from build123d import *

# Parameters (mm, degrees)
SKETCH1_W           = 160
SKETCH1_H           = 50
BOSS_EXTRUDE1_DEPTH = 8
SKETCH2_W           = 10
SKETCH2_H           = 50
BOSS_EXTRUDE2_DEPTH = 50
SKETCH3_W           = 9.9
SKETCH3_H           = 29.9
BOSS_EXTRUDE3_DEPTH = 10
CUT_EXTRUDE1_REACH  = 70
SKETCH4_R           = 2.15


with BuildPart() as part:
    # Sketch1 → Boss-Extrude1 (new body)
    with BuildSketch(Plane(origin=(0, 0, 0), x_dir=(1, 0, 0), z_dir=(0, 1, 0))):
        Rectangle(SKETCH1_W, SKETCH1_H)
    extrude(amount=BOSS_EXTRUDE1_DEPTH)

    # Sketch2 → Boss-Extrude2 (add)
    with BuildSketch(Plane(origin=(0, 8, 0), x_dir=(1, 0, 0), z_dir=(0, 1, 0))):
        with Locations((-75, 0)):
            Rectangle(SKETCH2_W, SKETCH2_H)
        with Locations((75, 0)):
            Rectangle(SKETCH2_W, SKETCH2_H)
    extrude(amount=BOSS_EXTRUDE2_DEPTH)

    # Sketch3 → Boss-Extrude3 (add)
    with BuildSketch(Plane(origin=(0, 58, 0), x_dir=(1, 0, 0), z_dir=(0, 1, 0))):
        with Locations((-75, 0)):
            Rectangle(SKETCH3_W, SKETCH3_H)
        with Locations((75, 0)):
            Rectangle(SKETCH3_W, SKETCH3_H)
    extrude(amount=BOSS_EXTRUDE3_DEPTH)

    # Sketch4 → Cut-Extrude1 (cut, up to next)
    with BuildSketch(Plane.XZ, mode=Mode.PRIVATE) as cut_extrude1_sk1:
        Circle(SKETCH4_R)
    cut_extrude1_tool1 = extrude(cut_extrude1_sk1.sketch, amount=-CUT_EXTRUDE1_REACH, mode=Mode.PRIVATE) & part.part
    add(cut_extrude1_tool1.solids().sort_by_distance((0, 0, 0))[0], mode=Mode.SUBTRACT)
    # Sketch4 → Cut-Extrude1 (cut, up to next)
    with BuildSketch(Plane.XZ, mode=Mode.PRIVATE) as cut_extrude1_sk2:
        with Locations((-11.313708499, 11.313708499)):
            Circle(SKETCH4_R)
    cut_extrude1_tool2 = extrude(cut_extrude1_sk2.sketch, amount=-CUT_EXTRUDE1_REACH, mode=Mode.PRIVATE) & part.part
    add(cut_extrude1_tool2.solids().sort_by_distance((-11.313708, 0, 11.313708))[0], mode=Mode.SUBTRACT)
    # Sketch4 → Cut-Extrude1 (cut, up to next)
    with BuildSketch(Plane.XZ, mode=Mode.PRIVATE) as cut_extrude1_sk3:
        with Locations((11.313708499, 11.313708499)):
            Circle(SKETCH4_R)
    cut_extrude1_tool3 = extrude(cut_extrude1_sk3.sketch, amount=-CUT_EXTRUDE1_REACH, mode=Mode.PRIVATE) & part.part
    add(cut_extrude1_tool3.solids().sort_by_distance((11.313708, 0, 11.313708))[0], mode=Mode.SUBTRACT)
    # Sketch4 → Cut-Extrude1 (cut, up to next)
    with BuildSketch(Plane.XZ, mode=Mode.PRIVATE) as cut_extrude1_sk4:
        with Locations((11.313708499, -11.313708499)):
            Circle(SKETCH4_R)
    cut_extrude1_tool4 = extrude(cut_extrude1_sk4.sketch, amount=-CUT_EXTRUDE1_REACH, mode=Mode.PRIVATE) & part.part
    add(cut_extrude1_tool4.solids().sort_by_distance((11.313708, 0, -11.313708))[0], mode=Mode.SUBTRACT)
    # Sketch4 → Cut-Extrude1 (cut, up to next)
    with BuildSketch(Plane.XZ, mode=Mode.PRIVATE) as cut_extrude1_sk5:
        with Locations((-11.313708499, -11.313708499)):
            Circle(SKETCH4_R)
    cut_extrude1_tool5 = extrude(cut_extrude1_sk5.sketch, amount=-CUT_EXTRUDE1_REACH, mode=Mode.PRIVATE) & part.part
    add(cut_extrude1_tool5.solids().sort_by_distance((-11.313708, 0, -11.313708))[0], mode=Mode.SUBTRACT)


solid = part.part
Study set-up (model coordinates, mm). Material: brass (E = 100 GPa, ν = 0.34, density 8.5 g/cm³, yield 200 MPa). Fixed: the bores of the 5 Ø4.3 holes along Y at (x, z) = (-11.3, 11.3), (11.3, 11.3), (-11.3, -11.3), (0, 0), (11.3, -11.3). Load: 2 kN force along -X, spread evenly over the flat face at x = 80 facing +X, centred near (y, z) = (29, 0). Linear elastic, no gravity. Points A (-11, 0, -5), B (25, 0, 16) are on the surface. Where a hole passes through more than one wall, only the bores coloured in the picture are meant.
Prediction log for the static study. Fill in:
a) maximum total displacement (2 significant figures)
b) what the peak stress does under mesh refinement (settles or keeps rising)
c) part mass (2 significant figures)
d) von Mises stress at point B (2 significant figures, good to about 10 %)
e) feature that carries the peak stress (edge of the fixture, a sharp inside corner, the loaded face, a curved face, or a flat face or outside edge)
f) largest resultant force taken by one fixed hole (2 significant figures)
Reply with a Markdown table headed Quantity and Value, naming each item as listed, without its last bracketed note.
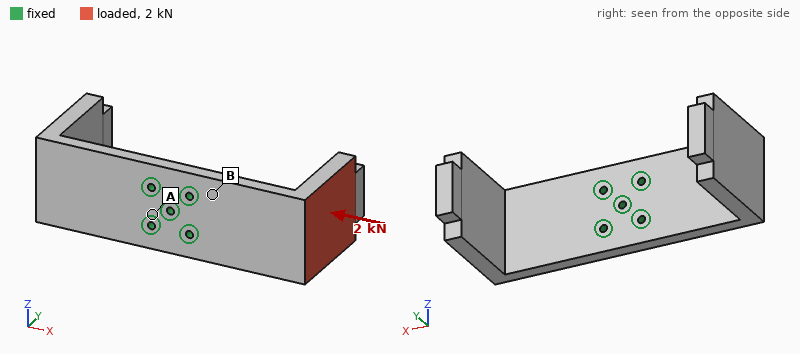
| Quantity | Value |
|---|---|
| maximum total displacement | 1.1 mm |
| what the peak stress does under mesh refinement | keeps rising |
| part mass | 1.0 kg |
| von Mises stress at point B | 84 MPa |
| feature that carries the peak stress | edge of the fixture |
| largest resultant force taken by one fixed hole | 920 N |
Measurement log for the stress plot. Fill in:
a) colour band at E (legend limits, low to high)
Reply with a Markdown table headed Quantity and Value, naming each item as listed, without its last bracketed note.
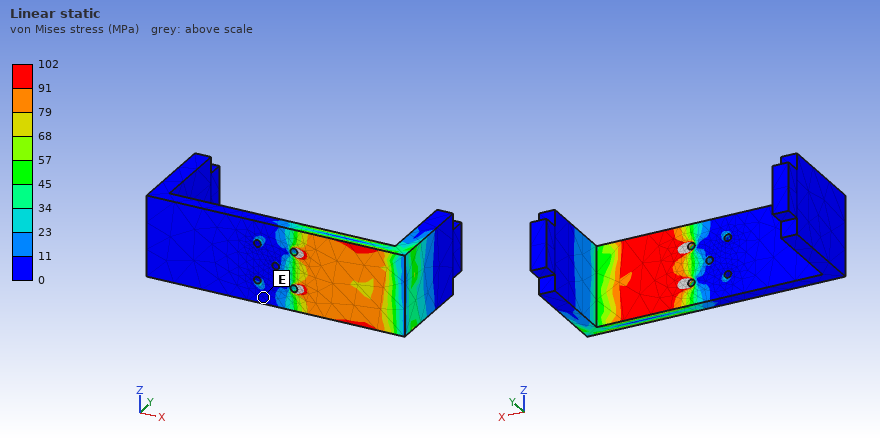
| Quantity | Value |
|---|---|
| colour band at E | 0 to 11 MPa |
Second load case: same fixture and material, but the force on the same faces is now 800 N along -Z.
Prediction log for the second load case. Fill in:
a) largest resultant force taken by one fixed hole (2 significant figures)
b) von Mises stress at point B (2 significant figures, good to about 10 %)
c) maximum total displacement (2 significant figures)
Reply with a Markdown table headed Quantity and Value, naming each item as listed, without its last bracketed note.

| Quantity | Value |
|---|---|
| largest resultant force taken by one fixed hole | 1.7 kN |
| von Mises stress at point B | 28 MPa |
| maximum total displacement | 0.22 mm |
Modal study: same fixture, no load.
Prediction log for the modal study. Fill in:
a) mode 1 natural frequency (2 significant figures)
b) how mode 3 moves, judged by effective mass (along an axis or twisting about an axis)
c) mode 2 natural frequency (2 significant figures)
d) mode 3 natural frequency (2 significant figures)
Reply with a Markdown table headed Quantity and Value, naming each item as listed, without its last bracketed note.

| Quantity | Value |
|---|---|
| mode 1 natural frequency | 350 Hz |
| how mode 3 moves, judged by effective mass | twisting about Y |
| mode 2 natural frequency | 350 Hz |
| mode 3 natural frequency | 630 Hz |
